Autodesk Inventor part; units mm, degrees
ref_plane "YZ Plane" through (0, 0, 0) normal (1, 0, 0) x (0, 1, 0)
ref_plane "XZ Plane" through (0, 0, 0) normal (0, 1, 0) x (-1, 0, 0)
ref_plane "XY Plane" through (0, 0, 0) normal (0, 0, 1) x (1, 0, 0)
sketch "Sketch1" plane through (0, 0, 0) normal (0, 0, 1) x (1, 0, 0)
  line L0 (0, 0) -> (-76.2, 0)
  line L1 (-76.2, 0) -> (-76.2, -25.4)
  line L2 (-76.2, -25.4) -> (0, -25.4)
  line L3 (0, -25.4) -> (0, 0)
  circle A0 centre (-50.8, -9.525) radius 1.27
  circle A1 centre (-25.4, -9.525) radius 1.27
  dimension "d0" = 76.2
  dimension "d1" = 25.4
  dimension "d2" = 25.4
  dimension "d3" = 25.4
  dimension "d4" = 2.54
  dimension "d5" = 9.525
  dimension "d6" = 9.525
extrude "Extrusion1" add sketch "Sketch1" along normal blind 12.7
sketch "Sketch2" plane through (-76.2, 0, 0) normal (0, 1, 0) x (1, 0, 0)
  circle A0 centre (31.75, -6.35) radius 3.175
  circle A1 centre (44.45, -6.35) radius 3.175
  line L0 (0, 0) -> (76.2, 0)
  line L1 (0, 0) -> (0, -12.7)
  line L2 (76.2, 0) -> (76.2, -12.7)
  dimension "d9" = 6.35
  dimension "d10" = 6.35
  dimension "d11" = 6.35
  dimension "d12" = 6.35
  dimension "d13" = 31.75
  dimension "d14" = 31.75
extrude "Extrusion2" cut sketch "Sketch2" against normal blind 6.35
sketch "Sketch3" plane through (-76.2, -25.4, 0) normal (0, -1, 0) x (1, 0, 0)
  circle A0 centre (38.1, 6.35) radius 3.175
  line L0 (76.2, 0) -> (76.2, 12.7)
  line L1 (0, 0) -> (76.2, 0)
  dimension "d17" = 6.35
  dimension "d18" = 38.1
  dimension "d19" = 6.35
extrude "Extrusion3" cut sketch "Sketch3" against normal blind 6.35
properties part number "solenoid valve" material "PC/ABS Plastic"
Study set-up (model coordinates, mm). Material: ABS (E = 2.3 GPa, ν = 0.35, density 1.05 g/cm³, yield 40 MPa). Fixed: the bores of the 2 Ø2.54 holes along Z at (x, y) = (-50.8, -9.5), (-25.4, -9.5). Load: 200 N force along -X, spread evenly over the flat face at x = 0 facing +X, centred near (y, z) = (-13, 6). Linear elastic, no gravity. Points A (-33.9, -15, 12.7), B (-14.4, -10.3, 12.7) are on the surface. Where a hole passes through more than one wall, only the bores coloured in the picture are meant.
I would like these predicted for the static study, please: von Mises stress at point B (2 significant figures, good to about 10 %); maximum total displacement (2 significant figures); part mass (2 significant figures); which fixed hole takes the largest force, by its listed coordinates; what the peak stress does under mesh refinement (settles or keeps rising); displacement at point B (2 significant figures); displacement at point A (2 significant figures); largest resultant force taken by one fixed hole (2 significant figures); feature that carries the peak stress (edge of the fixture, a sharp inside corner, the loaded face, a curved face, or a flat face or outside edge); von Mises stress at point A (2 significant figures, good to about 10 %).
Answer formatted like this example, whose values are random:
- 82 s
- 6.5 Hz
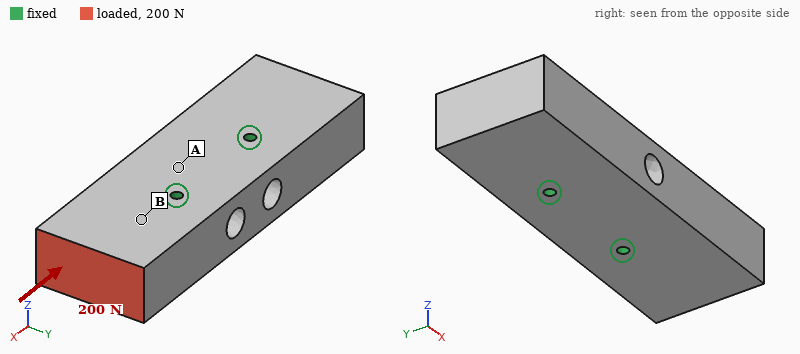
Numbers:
- 0.78 MPa
- 14 µm
- 25 g
- (-25.4, -9.5)
- keeps rising
- 5.5 µm
- 2.2 µm
- 160 N
- edge of the fixture
- 0.35 MPa
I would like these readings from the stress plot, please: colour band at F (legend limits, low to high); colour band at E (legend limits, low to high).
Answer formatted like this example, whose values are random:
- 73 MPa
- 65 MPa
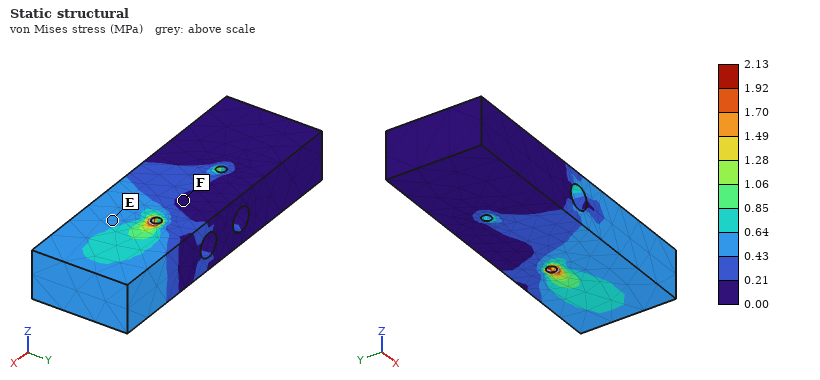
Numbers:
- 0.00 to 0.21 MPa
- 0.43 to 0.64 MPa
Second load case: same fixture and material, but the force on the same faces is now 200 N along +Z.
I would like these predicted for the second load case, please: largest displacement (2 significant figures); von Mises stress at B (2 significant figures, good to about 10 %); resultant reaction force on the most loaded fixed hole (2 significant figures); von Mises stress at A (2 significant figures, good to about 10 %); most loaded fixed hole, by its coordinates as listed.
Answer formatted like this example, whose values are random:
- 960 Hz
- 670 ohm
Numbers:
- 0.21 mm
- 4.5 MPa
- 280 N
- 2.4 MPa
- (-25.4, -9.5)
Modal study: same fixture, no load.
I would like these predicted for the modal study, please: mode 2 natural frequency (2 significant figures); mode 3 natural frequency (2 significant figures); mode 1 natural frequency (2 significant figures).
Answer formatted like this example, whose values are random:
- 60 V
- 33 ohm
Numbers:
- 3200 Hz
- 3500 Hz
- 3100 Hz
